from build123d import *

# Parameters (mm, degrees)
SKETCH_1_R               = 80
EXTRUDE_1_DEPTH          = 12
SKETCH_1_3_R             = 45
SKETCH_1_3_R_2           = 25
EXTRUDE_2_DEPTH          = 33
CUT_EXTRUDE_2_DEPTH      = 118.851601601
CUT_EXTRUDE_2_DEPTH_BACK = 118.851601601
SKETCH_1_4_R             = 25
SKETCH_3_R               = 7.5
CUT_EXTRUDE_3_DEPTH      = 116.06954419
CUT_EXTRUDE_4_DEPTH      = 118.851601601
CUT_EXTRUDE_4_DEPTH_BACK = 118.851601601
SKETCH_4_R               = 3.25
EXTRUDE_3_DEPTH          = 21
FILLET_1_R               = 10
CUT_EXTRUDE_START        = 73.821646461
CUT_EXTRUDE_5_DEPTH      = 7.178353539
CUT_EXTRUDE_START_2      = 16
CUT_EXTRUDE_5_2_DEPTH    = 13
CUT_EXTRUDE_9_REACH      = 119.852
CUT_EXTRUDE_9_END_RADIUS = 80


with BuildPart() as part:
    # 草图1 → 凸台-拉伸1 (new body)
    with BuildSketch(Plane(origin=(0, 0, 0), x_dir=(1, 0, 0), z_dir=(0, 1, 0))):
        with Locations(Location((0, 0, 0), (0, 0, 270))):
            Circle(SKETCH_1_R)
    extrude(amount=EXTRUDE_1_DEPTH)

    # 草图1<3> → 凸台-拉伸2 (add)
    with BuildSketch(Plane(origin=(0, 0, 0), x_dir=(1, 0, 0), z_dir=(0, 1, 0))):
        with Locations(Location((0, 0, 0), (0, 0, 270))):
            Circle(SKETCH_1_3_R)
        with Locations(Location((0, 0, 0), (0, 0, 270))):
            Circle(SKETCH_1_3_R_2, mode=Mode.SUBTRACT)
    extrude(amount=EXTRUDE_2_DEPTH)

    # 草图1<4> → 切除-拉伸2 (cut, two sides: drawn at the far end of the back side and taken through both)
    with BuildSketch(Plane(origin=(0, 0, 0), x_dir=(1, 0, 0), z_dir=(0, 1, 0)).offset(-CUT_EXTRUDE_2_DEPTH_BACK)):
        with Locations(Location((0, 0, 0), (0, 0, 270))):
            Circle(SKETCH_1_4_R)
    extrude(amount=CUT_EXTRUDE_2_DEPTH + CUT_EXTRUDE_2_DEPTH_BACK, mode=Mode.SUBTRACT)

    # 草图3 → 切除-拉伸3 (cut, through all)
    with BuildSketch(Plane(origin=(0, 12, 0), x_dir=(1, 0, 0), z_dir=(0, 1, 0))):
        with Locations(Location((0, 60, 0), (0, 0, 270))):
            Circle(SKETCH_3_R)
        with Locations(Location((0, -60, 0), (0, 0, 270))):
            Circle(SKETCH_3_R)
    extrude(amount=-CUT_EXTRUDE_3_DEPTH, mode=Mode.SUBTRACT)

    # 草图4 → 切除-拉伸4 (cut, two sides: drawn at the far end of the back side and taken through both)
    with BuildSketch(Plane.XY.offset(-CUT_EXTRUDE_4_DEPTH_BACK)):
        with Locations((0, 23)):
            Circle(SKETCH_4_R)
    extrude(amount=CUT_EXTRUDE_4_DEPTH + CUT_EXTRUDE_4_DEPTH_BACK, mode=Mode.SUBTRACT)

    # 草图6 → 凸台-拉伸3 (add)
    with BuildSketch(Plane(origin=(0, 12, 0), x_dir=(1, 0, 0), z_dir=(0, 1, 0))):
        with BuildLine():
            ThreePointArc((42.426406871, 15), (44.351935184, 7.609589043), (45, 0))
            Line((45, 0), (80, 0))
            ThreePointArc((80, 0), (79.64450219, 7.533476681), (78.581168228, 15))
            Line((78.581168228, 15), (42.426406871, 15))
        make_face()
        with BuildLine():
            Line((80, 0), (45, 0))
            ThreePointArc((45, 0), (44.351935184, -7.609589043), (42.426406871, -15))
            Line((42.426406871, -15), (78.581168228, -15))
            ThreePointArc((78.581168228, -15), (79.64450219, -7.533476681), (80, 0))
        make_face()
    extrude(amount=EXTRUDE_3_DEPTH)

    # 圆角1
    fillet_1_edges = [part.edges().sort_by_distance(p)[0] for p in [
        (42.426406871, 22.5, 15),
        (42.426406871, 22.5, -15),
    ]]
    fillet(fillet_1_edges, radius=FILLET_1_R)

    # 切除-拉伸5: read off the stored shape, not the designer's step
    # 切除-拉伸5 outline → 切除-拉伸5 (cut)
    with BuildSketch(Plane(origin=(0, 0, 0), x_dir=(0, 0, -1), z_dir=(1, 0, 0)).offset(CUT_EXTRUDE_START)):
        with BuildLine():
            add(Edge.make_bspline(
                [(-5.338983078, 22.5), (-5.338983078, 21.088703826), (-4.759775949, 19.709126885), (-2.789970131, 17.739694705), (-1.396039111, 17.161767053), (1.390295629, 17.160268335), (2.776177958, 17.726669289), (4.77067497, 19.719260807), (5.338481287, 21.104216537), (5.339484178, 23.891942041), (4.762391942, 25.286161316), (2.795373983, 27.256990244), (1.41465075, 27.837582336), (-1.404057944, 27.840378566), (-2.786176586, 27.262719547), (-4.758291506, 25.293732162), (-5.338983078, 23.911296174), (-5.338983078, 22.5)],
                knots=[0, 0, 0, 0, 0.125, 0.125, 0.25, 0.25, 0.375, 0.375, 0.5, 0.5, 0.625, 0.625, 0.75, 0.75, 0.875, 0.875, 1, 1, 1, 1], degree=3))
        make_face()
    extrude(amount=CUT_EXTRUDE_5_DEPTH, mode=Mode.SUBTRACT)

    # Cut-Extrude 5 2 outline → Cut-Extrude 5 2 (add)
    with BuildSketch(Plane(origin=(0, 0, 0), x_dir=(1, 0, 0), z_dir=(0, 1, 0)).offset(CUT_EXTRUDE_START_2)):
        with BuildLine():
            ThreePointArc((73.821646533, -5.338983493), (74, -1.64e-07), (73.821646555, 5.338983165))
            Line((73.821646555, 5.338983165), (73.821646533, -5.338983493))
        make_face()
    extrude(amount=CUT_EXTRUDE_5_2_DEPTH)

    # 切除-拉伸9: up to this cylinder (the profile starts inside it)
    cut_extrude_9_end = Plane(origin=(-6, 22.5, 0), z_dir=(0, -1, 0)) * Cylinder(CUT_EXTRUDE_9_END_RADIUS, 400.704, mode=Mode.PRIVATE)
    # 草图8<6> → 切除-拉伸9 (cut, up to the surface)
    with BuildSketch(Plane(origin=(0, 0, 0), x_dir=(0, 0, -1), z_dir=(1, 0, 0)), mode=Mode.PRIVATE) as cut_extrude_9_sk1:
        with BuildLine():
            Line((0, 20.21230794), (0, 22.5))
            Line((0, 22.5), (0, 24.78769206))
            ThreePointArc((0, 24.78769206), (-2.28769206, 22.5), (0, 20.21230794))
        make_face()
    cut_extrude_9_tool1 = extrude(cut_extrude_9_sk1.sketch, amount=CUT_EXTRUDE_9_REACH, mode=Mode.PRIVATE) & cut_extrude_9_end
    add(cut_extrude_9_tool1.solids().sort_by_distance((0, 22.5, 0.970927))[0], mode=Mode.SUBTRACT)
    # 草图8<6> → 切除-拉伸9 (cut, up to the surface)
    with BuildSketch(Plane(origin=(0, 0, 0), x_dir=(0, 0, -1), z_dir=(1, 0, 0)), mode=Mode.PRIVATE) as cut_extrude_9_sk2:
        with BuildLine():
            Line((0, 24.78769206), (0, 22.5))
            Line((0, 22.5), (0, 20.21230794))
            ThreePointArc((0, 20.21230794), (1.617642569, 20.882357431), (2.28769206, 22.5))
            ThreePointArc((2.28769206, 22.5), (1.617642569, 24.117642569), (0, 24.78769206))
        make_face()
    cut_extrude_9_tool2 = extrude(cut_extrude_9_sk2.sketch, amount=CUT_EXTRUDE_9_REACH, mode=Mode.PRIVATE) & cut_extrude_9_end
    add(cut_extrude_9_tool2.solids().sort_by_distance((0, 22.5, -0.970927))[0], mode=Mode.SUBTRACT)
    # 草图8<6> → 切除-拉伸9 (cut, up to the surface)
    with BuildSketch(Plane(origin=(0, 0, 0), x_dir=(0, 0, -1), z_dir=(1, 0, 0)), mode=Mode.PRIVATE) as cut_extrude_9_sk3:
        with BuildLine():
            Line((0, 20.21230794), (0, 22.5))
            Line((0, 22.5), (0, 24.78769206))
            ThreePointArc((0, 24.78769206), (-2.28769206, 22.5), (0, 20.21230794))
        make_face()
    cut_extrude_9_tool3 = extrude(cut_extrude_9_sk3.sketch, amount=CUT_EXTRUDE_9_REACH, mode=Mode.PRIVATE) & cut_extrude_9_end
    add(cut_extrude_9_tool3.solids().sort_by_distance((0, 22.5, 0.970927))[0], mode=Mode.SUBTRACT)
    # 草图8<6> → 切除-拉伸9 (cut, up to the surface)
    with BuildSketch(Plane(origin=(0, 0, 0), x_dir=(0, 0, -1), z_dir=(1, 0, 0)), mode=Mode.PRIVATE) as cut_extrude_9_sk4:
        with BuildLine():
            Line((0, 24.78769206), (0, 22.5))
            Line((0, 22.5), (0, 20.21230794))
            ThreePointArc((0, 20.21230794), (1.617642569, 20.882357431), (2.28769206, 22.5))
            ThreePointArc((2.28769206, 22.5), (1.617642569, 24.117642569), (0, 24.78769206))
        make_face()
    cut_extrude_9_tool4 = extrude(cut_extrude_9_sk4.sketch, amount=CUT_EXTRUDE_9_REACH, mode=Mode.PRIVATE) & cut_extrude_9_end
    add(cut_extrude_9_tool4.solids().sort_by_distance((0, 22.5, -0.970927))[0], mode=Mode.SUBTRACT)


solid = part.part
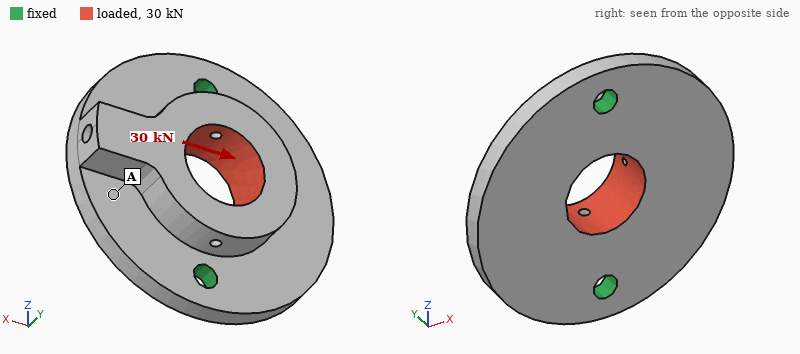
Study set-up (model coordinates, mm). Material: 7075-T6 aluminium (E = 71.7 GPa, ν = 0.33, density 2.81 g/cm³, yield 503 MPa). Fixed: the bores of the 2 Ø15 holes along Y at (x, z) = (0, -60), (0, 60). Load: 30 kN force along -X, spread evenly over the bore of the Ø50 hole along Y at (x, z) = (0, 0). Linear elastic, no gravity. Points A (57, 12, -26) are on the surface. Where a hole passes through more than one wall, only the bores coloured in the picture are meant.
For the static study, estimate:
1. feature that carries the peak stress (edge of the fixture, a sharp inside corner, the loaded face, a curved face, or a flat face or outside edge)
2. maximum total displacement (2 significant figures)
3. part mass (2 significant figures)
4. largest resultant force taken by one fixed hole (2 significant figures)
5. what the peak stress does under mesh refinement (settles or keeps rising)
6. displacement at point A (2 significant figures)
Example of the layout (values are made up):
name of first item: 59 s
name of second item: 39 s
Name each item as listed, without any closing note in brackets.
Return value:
feature that carries the peak stress: edge of the fixture
maximum total displacement: 0.21 mm
part mass: 920 g
largest resultant force taken by one fixed hole: 15 kN
what the peak stress does under mesh refinement: keeps rising
displacement at point A: 0.13 mm
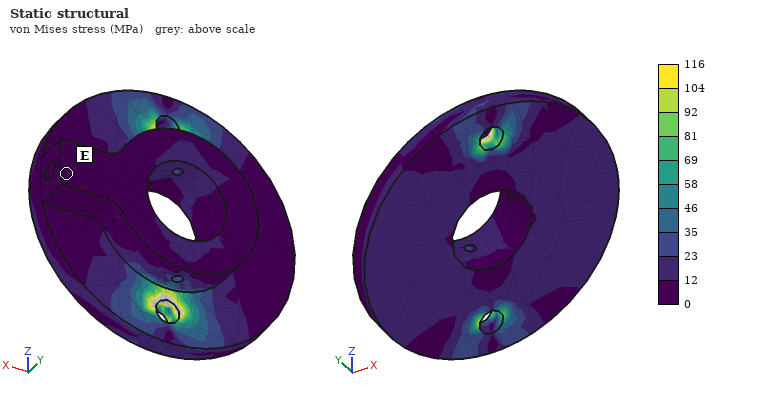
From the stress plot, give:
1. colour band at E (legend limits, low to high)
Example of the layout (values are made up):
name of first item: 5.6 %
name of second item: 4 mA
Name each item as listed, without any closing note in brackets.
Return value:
colour band at E: 0 to 12 MPa
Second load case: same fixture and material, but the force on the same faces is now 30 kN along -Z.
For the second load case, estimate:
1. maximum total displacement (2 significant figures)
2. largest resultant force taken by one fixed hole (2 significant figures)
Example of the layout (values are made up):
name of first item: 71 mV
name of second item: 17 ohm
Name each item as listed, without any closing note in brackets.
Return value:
maximum total displacement: 20 µm
largest resultant force taken by one fixed hole: 15 kN
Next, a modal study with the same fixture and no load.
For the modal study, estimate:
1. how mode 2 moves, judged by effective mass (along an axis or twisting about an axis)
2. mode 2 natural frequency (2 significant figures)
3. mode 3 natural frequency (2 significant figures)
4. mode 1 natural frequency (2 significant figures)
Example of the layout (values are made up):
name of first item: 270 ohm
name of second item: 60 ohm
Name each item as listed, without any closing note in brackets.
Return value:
how mode 2 moves, judged by effective mass: along Y
mode 2 natural frequency: 2700 Hz
mode 3 natural frequency: 5200 Hz
mode 1 natural frequency: 1500 Hz
